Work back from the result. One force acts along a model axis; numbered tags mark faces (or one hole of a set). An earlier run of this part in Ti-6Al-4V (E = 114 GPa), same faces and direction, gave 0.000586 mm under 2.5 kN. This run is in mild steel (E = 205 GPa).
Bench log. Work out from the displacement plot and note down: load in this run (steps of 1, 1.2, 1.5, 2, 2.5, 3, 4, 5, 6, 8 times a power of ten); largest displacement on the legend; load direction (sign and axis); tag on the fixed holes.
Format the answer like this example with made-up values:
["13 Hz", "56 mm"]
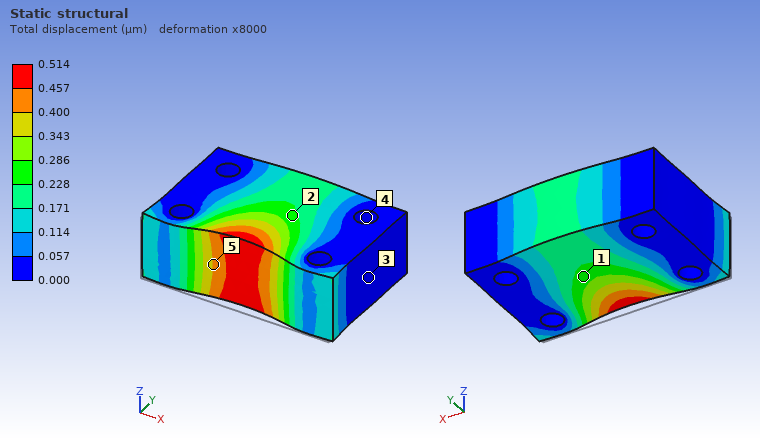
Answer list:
["4 kN", "0.514 µm", "+Y", "4"]
